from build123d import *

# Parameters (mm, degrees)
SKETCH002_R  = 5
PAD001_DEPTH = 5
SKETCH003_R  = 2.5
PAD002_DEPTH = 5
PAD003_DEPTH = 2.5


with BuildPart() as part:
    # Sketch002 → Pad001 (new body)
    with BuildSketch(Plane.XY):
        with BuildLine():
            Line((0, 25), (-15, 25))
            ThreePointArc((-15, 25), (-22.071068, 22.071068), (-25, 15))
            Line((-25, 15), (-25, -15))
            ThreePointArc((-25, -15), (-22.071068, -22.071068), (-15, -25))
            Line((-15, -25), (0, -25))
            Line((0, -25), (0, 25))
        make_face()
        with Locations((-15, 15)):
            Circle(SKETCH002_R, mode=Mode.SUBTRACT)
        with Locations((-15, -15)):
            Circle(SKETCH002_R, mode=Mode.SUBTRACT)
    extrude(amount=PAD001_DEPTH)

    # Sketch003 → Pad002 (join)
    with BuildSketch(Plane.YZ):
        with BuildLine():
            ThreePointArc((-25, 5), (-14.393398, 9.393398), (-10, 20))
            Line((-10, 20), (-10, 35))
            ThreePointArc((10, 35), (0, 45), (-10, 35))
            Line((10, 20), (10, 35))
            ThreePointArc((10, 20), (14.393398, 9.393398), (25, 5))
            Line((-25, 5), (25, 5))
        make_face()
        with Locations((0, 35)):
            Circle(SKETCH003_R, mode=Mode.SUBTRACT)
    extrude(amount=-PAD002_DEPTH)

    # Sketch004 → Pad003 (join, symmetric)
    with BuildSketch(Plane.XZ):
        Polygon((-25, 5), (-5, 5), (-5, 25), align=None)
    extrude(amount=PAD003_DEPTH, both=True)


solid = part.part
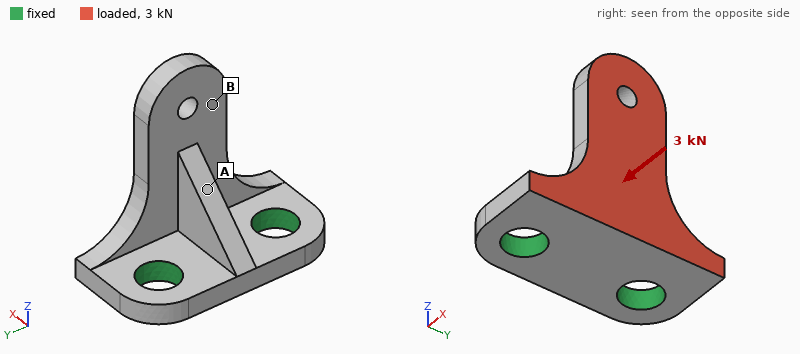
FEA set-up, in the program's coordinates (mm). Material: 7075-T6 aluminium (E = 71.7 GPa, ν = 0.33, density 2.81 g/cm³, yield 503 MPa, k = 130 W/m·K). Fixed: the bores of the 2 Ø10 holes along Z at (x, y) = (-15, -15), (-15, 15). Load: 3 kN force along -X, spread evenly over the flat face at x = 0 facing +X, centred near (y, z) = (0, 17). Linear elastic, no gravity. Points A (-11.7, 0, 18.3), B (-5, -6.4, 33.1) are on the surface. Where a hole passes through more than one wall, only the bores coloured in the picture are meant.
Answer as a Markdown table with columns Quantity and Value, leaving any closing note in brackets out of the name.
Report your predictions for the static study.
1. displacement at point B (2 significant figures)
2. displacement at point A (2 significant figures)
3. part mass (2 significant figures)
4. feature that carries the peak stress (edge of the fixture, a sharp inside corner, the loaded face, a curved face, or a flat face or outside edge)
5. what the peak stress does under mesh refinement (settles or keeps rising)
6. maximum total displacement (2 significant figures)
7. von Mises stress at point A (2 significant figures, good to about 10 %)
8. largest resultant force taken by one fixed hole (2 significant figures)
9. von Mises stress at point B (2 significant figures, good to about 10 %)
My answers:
| Quantity | Value |
|---|---|
| displacement at point B | 0.22 mm |
| displacement at point A | 0.076 mm |
| part mass | 29 g |
| feature that carries the peak stress | edge of the fixture |
| what the peak stress does under mesh refinement | keeps rising |
| maximum total displacement | 0.37 mm |
| von Mises stress at point A | 120 MPa |
| largest resultant force taken by one fixed hole | 1.5 kN |
| von Mises stress at point B | 36 MPa |
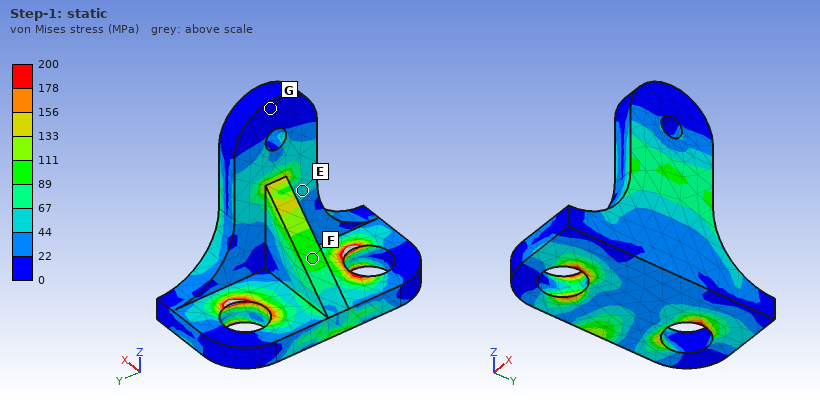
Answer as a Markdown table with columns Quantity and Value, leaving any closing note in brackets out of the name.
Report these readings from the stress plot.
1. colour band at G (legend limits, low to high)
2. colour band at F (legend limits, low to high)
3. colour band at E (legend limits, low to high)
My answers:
| Quantity | Value |
|---|---|
| colour band at G | 0 to 22 MPa |
| colour band at F | 89 to 111 MPa |
| colour band at E | 44 to 67 MPa |
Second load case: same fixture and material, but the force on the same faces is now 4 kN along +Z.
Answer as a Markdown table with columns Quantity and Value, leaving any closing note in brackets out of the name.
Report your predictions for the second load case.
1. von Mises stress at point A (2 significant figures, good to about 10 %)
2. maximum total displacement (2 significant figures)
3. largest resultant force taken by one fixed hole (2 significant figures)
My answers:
| Quantity | Value |
|---|---|
| von Mises stress at point A | 35 MPa |
| maximum total displacement | 0.24 mm |
| largest resultant force taken by one fixed hole | 2.1 kN |
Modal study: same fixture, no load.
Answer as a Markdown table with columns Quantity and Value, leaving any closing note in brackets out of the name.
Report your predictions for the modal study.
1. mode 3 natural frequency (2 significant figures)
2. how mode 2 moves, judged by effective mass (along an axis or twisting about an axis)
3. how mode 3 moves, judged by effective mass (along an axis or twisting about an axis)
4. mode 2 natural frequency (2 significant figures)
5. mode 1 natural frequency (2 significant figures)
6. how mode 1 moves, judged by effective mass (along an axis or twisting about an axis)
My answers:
| Quantity | Value |
|---|---|
| mode 3 natural frequency | 12 kHz |
| how mode 2 moves, judged by effective mass | along Y |
| how mode 3 moves, judged by effective mass | along Z |
| mode 2 natural frequency | 8300 Hz |
| mode 1 natural frequency | 4700 Hz |
| how mode 1 moves, judged by effective mass | along X |
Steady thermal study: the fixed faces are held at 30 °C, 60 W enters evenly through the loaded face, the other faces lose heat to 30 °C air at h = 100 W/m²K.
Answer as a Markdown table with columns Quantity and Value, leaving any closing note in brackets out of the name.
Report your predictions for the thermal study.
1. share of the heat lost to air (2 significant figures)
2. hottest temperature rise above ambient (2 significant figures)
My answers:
| Quantity | Value |
|---|---|
| share of the heat lost to air | 12 % |
| hottest temperature rise above ambient | 56 K |
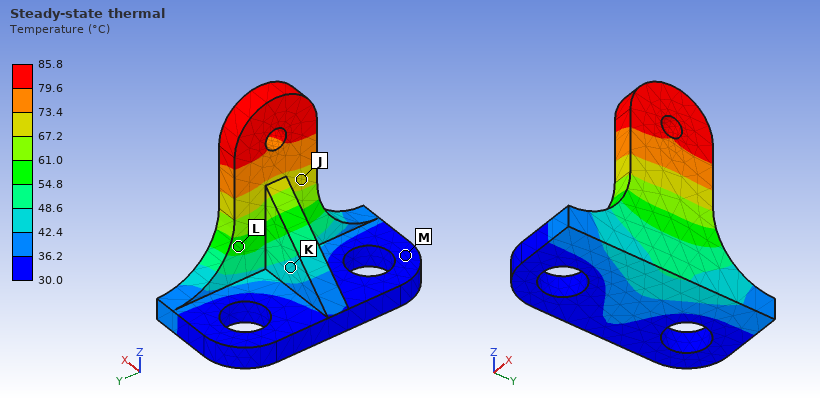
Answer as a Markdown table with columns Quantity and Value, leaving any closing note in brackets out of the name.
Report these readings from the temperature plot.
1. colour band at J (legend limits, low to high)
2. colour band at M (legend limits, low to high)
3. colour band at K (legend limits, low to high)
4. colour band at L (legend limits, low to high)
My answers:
| Quantity | Value |
|---|---|
| colour band at J | 67.2 to 73.4 °C |
| colour band at M | 30.0 to 36.2 °C |
| colour band at K | 42.4 to 48.6 °C |
| colour band at L | 54.8 to 61.0 °C |
